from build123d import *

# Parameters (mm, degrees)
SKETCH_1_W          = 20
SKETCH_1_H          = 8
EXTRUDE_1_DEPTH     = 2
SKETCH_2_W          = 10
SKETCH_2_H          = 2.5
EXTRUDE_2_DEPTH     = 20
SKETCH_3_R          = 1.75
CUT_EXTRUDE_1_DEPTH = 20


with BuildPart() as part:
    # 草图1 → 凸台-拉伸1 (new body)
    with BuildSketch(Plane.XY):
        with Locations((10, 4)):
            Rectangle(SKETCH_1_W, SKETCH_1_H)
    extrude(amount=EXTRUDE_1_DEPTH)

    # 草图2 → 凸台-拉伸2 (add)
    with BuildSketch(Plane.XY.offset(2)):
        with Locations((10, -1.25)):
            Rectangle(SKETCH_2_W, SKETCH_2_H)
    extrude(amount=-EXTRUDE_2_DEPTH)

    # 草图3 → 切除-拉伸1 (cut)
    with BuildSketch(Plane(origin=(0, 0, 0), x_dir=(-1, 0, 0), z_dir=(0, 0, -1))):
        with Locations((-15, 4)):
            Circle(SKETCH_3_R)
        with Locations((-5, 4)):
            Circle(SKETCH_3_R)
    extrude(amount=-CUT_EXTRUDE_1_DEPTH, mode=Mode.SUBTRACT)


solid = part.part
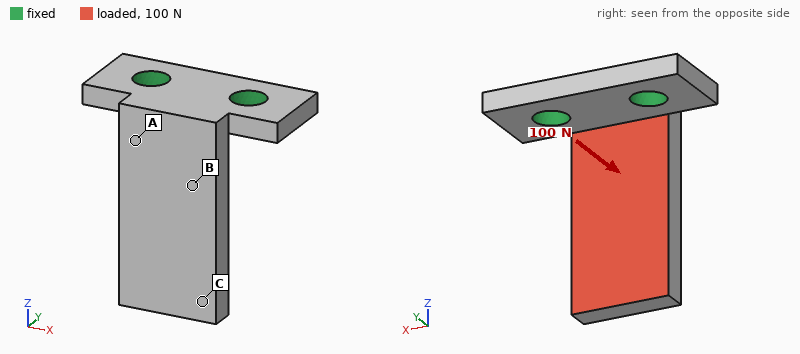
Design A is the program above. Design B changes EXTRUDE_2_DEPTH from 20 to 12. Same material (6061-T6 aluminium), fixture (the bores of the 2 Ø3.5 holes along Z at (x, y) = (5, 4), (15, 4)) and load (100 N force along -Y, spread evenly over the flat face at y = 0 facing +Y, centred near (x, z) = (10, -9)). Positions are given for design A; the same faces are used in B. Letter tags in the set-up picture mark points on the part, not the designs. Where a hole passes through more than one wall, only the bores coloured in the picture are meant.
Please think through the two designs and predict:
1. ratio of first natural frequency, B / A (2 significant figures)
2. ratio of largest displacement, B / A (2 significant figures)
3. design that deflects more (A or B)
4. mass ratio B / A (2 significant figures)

2.4
0.29
A
0.74
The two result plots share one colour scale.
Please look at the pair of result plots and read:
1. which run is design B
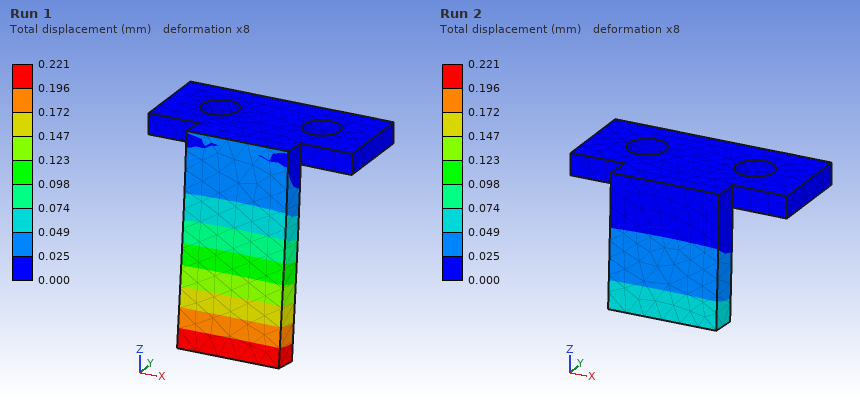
Run 2
